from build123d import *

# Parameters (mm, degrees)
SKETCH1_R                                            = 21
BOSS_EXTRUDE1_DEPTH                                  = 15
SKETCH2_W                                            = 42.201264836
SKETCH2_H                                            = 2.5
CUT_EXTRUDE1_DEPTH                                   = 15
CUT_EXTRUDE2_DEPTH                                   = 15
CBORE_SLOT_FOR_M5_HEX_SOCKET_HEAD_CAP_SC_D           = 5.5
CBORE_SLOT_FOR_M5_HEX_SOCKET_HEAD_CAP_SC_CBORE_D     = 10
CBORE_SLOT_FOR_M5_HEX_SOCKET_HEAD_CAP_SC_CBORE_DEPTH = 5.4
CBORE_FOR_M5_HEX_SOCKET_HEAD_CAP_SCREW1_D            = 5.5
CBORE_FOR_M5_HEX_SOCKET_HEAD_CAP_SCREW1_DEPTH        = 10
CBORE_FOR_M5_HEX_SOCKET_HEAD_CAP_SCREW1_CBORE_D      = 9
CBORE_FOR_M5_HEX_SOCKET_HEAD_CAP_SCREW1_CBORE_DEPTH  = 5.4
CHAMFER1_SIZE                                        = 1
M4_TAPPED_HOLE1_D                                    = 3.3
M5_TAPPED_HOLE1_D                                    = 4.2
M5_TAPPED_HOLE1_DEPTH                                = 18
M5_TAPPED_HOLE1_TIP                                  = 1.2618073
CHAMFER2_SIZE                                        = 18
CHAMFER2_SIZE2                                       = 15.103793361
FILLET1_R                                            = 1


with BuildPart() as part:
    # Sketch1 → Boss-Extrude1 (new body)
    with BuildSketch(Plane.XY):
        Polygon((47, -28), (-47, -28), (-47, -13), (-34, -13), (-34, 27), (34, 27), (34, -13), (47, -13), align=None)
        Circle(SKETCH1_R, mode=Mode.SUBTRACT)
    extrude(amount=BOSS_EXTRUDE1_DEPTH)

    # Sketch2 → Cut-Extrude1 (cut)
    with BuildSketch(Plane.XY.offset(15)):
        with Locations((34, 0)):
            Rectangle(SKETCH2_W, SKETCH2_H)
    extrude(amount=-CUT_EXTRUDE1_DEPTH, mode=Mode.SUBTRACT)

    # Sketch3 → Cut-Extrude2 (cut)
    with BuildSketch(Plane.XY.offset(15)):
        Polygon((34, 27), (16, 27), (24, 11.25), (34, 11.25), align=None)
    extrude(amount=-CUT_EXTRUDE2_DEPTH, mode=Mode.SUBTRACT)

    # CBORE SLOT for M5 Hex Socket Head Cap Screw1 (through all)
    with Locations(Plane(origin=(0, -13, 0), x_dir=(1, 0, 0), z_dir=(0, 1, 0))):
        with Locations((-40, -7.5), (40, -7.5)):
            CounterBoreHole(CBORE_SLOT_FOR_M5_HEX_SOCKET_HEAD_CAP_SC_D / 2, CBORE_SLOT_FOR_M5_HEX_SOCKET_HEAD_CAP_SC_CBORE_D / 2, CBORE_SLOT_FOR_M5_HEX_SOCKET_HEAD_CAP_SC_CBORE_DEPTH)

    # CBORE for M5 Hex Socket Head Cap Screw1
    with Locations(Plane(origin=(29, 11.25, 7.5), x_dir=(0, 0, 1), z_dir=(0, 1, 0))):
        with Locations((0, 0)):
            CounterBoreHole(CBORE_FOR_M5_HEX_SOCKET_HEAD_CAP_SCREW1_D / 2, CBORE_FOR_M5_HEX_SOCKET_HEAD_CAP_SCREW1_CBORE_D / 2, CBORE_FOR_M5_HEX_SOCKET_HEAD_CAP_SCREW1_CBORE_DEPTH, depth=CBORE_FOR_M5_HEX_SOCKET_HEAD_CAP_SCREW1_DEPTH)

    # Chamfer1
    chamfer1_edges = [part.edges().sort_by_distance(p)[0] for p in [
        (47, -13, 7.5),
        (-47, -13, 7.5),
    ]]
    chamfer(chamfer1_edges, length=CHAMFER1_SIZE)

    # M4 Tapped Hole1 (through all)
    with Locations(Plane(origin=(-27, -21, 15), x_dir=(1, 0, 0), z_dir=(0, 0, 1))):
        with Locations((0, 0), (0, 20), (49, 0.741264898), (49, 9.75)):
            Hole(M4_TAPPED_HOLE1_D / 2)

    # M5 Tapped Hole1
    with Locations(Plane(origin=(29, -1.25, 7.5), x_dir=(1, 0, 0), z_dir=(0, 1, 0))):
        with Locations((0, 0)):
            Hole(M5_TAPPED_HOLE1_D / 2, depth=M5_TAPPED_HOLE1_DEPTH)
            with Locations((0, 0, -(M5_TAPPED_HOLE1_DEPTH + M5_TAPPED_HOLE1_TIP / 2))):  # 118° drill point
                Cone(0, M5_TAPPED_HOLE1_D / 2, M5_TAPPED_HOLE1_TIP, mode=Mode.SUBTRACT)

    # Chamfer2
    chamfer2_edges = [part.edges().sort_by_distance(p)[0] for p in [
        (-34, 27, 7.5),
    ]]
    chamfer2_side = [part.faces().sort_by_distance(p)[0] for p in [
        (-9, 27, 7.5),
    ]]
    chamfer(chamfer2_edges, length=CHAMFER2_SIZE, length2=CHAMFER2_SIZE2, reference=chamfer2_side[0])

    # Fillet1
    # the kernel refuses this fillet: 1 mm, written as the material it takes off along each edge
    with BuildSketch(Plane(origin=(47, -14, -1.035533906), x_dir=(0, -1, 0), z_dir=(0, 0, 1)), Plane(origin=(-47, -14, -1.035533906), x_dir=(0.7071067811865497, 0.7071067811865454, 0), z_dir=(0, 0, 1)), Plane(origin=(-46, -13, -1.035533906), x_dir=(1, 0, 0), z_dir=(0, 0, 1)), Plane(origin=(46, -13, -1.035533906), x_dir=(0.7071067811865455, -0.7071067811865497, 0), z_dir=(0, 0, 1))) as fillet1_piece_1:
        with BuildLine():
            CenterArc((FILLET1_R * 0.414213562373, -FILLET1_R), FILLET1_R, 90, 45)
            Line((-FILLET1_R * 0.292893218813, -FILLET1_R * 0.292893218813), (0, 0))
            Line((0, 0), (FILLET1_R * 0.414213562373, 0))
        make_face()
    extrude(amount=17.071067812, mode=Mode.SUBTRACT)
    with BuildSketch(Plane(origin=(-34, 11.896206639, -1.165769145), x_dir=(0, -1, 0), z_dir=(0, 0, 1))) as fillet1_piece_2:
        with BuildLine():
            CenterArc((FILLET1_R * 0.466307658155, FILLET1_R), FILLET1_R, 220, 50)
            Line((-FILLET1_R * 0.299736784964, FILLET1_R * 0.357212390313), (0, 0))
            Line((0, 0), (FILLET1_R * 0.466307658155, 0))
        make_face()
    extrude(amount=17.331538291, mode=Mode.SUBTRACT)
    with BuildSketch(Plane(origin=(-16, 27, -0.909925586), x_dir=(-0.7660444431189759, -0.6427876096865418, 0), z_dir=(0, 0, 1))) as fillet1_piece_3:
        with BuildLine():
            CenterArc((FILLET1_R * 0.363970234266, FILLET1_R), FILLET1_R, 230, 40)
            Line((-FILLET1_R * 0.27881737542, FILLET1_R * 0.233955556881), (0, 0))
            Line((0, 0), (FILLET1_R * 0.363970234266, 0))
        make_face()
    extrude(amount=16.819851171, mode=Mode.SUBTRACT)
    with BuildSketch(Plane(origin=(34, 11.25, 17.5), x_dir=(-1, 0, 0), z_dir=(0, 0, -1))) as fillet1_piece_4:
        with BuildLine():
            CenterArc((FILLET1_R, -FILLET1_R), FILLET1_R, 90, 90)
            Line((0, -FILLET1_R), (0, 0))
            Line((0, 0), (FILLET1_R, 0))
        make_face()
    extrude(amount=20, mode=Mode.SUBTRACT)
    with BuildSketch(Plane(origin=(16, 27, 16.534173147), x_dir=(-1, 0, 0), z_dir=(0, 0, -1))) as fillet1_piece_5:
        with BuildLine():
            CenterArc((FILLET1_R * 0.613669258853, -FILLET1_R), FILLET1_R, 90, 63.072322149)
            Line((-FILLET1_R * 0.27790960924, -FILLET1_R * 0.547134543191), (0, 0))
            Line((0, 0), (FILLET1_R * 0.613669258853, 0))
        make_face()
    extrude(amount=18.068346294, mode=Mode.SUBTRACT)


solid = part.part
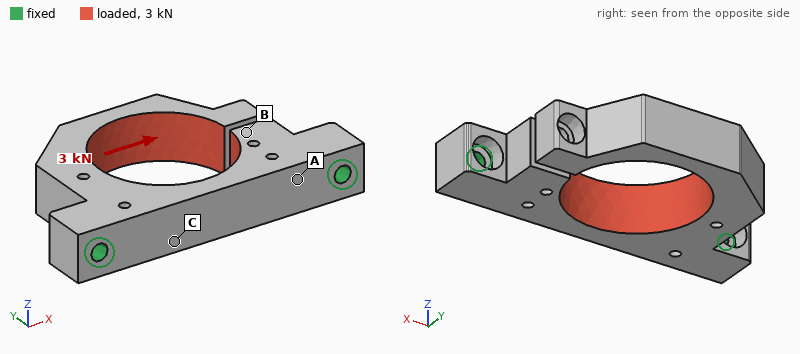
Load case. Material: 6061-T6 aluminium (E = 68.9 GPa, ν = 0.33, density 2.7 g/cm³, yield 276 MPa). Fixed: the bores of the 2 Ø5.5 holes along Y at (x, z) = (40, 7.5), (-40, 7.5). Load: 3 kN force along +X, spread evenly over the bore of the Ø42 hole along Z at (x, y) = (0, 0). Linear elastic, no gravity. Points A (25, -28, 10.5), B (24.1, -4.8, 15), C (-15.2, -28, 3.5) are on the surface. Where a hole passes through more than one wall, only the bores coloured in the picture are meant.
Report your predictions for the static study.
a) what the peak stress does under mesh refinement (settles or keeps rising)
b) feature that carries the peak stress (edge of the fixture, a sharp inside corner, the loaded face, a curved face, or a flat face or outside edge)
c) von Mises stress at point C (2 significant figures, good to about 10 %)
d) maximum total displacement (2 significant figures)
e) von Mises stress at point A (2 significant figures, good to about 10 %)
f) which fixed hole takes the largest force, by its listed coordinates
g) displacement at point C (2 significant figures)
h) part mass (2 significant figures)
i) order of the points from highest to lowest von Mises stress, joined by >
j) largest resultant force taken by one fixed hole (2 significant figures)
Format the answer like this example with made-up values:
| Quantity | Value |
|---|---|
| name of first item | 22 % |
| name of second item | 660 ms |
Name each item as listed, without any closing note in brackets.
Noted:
| Quantity | Value |
|---|---|
| what the peak stress does under mesh refinement | keeps rising |
| feature that carries the peak stress | edge of the fixture |
| von Mises stress at point C | 47 MPa |
| maximum total displacement | 0.29 mm |
| von Mises stress at point A | 16 MPa |
| which fixed hole takes the largest force, by its listed coordinates | (-40, 7.5) |
| displacement at point C | 0.047 mm |
| part mass | 89 g |
| order of the points from highest to lowest von Mises stress, joined by > | C > A > B |
| largest resultant force taken by one fixed hole | 2.7 kN |
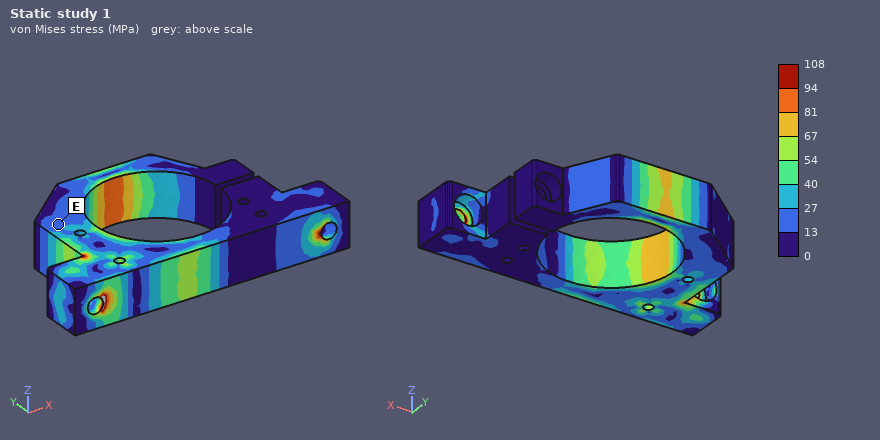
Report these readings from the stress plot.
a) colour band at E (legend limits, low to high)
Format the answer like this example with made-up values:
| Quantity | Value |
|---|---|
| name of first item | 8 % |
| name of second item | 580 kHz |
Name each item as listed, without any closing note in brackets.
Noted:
| Quantity | Value |
|---|---|
| colour band at E | 13 to 27 MPa |
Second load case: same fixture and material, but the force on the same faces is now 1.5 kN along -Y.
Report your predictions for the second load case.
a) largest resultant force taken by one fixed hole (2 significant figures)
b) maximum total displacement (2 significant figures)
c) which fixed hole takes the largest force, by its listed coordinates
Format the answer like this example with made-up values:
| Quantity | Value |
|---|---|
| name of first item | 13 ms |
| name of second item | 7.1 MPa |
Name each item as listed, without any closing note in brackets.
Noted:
| Quantity | Value |
|---|---|
| largest resultant force taken by one fixed hole | 930 N |
| maximum total displacement | 0.57 mm |
| which fixed hole takes the largest force, by its listed coordinates | (-40, 7.5) |
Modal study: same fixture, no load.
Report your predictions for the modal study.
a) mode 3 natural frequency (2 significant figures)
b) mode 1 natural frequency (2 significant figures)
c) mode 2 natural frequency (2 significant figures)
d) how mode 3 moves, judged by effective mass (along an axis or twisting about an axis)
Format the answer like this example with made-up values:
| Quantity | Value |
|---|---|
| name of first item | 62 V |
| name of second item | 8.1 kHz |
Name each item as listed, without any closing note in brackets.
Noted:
| Quantity | Value |
|---|---|
| mode 3 natural frequency | 2500 Hz |
| mode 1 natural frequency | 1300 Hz |
| mode 2 natural frequency | 1400 Hz |
| how mode 3 moves, judged by effective mass | along X |
